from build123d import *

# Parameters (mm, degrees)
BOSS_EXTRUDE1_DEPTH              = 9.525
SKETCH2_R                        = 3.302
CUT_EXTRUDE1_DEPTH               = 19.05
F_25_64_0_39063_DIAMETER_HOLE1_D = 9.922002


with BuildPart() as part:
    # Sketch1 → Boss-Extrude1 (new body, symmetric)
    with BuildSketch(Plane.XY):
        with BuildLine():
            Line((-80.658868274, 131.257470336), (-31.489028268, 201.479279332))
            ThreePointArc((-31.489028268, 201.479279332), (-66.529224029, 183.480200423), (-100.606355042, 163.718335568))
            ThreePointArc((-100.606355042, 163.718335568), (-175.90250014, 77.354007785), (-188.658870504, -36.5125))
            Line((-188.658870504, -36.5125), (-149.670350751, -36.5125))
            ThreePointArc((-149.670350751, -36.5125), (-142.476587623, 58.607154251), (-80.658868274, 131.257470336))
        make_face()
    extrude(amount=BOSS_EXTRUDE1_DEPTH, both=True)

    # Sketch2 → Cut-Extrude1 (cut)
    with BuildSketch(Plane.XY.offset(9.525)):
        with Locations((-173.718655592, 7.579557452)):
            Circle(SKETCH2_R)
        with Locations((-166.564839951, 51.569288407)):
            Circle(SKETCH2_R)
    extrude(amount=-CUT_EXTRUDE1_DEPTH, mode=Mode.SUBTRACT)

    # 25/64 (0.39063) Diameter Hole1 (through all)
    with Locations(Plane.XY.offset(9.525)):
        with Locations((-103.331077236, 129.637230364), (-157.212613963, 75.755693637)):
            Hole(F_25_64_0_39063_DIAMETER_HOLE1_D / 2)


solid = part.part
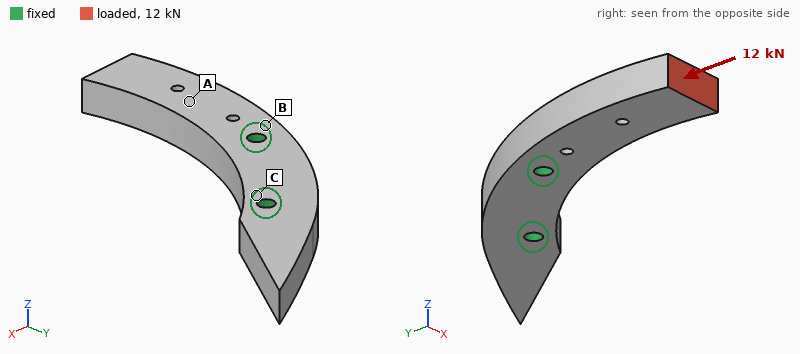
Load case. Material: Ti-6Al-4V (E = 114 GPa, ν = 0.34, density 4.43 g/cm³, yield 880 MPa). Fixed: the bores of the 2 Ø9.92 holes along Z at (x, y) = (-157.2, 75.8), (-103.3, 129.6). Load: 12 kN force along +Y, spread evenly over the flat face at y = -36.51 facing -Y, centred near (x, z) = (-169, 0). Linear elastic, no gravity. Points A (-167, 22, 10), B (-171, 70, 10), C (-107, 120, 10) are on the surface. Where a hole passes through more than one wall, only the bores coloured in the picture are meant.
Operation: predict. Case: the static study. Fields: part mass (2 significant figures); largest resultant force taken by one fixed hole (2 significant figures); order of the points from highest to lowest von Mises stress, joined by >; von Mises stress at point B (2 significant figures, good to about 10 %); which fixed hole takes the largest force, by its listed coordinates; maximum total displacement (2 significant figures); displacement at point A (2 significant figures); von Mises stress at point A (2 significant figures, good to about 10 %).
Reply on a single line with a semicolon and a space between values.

800 g; 12 kN; B > A > C; 27 MPa; (-157.2, 75.8); 64 µm; 32 µm; 18 MPa
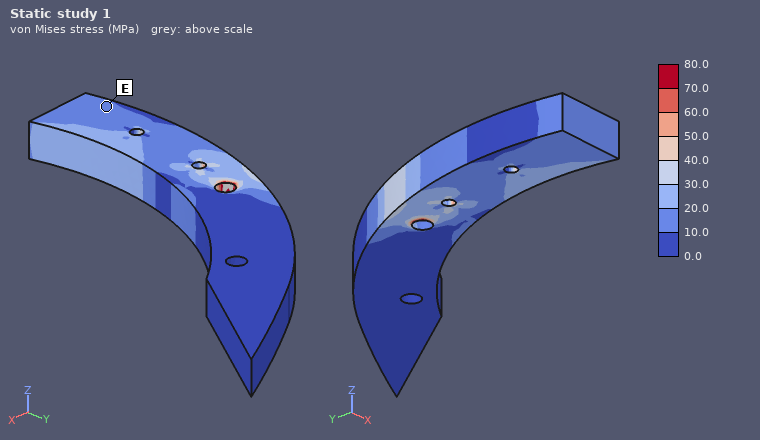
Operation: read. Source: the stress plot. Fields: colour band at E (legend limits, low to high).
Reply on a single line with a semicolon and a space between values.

10.0 to 20.0 MPa
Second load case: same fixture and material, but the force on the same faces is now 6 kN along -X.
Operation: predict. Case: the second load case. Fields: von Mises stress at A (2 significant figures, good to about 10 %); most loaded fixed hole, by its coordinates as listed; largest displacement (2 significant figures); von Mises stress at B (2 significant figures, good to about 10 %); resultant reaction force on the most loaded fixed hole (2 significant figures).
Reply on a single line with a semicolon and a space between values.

28 MPa; (-157.2, 75.8); 0.45 mm; 80 MPa; 11 kN
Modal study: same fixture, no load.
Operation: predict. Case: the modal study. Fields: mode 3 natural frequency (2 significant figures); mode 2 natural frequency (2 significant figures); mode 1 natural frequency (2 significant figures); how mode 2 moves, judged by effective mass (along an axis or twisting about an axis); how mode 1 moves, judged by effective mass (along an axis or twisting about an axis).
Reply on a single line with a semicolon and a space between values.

2700 Hz; 1800 Hz; 1200 Hz; along X; along Z
